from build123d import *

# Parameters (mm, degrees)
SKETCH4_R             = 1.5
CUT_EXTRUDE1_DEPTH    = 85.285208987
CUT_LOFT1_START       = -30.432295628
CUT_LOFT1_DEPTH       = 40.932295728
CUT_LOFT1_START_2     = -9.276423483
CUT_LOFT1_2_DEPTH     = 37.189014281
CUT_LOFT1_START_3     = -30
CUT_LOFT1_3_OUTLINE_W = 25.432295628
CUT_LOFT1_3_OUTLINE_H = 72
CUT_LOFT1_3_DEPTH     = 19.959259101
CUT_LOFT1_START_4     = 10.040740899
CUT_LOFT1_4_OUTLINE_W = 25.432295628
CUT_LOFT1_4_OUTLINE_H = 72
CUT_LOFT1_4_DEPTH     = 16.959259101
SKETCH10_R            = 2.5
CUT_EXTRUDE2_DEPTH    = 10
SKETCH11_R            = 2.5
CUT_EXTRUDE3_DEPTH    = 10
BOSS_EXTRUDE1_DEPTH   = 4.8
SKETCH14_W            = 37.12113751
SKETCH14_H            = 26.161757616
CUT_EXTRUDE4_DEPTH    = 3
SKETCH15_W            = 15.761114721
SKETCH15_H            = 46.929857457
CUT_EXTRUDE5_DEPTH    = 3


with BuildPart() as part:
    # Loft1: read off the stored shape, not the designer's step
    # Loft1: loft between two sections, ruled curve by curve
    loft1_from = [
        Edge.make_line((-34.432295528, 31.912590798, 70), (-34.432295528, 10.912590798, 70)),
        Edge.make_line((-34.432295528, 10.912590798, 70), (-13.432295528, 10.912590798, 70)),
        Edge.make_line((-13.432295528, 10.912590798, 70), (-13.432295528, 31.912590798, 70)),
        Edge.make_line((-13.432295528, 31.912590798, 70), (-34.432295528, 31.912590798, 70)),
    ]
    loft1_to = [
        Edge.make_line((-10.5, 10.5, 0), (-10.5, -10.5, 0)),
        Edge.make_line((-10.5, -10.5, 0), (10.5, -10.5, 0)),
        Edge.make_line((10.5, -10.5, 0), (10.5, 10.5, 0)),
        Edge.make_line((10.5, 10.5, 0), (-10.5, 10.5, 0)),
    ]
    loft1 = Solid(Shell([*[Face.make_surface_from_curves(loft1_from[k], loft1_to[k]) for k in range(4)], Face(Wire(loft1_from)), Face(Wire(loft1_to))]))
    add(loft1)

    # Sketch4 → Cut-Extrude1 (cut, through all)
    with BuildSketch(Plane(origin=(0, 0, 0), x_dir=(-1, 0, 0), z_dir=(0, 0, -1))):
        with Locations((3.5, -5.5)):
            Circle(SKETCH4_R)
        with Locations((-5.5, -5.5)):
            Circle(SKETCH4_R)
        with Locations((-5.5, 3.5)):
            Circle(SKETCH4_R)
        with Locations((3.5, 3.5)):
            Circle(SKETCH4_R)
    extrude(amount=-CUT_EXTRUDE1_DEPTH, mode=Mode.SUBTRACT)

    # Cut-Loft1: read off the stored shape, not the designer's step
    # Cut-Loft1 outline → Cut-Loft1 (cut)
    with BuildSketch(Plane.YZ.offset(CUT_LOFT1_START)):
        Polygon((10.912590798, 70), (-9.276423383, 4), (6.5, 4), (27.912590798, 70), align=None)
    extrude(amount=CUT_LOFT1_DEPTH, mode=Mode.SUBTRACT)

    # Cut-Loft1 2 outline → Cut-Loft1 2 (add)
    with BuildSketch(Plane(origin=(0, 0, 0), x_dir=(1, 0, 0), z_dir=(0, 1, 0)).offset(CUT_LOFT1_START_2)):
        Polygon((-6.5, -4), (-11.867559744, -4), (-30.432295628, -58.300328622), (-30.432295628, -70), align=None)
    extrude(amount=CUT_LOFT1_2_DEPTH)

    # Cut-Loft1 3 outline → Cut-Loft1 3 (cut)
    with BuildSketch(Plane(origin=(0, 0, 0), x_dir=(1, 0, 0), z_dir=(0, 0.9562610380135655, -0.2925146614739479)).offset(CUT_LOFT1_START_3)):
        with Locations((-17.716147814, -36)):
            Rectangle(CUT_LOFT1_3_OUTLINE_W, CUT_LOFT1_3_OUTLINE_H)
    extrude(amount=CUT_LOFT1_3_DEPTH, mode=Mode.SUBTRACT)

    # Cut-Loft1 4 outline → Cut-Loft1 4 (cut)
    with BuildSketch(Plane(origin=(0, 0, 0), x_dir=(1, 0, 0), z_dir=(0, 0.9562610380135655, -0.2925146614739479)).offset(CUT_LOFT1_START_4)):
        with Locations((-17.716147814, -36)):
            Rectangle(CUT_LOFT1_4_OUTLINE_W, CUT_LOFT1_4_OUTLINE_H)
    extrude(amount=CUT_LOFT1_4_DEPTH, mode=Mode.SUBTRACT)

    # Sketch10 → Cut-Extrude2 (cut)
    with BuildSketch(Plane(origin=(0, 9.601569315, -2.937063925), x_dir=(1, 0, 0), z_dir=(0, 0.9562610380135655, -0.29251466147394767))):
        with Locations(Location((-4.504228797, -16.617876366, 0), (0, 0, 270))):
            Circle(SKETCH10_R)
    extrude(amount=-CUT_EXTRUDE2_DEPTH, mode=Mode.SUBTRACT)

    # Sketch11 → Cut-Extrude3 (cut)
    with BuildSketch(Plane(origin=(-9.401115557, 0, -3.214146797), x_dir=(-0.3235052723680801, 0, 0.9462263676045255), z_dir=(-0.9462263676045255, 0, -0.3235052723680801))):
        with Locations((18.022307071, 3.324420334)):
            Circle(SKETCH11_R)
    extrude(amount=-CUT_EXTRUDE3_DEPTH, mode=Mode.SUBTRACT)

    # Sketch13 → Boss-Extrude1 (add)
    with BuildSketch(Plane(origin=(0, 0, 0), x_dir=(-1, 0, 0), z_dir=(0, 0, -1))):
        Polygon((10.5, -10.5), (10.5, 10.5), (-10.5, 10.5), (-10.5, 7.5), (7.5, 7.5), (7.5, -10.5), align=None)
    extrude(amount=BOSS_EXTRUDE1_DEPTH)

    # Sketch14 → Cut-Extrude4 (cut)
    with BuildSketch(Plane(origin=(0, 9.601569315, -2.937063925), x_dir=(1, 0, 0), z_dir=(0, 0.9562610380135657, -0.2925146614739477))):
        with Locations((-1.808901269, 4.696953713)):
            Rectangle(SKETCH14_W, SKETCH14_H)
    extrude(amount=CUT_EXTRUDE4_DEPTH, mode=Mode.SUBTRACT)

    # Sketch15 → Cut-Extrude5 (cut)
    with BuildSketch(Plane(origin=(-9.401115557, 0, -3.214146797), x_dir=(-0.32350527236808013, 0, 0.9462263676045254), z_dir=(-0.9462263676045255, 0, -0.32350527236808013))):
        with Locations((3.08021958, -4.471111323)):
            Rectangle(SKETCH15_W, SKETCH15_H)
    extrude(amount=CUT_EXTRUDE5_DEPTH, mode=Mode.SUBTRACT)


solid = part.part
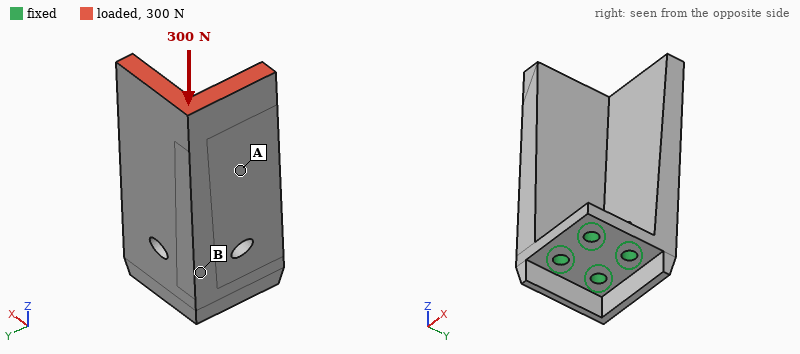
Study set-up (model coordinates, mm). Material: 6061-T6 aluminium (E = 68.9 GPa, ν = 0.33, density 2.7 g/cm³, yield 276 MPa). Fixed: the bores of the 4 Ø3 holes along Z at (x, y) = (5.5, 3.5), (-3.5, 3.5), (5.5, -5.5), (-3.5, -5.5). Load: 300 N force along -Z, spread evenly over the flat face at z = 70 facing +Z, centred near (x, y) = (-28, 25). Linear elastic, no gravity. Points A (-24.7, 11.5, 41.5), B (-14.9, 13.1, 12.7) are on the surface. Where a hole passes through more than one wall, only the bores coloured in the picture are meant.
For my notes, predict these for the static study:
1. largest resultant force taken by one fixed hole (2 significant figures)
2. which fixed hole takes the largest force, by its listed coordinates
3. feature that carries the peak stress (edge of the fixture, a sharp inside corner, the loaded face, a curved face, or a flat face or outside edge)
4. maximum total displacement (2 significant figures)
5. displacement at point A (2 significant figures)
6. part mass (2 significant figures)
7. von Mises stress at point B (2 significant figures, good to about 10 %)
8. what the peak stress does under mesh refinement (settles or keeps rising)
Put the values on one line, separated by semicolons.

1.3 kN; (-3.5, 3.5); edge of the fixture; 0.25 mm; 0.12 mm; 36 g; 27 MPa; keeps rising
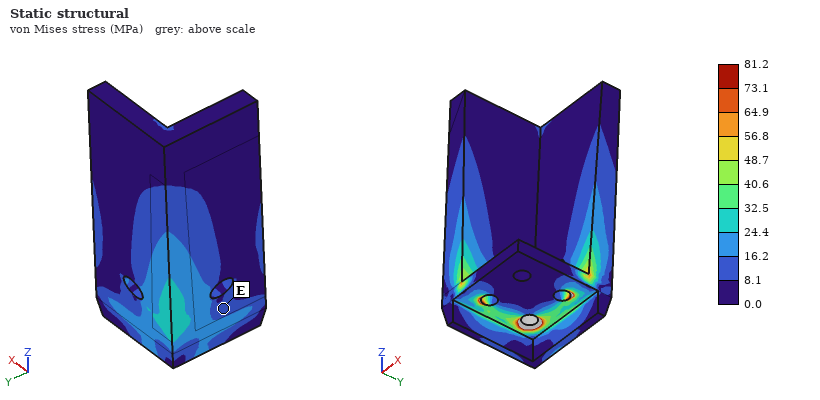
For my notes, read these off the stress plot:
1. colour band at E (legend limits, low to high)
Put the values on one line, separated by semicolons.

8.1 to 16.2 MPa
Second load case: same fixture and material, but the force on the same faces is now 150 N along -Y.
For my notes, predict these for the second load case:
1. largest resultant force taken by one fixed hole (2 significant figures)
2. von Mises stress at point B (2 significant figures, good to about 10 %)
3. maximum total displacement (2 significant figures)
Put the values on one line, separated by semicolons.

810 N; 19 MPa; 0.21 mm
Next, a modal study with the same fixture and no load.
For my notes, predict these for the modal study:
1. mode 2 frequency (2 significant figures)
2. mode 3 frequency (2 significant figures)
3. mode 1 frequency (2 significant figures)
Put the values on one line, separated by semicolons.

1900 Hz; 4100 Hz; 1300 Hz
